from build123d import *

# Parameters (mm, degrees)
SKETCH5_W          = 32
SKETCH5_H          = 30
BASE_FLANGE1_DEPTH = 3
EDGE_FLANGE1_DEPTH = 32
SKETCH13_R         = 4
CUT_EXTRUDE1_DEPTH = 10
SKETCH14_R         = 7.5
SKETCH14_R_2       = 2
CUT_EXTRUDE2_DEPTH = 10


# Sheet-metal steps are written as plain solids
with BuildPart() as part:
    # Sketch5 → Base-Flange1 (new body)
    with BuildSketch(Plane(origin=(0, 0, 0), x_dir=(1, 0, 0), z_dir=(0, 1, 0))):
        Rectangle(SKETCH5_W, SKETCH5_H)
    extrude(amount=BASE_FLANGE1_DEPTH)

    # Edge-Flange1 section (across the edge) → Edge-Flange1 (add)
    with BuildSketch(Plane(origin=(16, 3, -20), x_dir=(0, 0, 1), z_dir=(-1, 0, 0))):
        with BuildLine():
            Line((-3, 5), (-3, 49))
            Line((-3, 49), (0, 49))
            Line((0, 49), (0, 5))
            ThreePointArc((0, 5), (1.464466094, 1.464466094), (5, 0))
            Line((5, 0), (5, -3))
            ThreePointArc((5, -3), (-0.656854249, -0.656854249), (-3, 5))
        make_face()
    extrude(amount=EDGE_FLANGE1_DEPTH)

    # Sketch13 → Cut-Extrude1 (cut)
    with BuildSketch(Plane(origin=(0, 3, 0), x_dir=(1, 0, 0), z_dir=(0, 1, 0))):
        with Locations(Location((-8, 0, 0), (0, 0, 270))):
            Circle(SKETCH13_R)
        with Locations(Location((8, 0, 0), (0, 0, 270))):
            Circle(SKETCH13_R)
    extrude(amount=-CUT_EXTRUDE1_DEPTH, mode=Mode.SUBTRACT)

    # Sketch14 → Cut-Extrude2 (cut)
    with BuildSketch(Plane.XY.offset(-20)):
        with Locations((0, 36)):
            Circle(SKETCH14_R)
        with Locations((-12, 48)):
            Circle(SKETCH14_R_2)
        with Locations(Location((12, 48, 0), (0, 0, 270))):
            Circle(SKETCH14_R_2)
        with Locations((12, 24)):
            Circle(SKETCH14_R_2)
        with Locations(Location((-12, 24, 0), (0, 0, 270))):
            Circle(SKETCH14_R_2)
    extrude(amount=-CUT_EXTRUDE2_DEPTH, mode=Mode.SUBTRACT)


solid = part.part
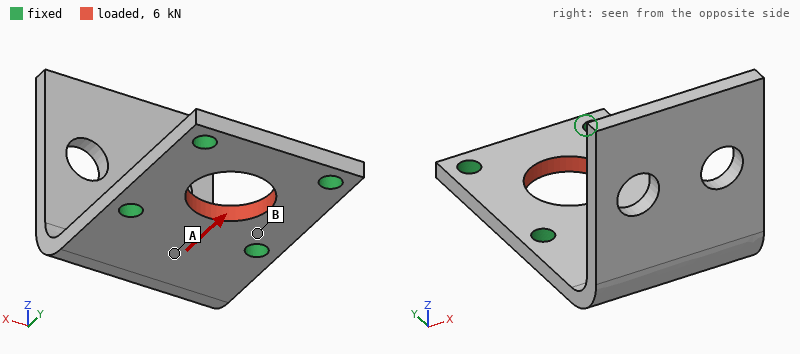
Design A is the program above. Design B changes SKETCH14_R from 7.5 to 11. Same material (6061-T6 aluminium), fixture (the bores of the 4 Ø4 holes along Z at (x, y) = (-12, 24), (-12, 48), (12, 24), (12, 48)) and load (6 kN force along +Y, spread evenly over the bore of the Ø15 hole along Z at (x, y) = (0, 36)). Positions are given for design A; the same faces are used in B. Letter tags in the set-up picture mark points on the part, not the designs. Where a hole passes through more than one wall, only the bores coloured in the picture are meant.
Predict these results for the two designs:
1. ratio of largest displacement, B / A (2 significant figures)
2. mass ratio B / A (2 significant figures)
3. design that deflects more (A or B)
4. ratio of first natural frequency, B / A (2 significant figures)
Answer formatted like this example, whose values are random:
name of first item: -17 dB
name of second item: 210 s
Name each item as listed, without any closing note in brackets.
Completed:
ratio of largest displacement, B / A: 1.4
mass ratio B / A: 0.91
design that deflects more: B
ratio of first natural frequency, B / A: 0.99
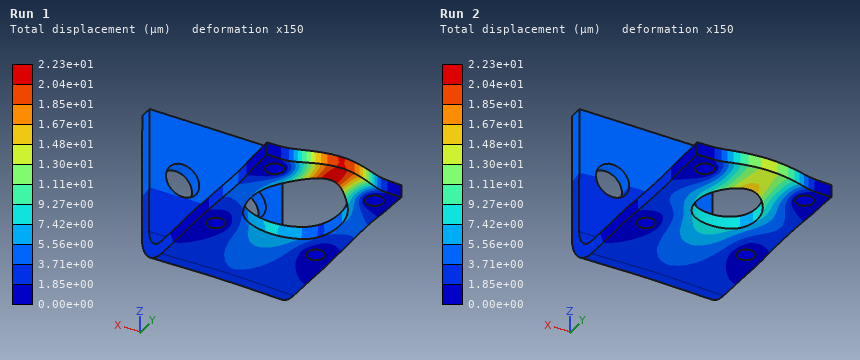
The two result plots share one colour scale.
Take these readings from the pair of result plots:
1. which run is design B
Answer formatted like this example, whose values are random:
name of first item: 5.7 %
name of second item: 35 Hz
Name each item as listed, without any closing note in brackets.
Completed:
which run is design B: Run 1
